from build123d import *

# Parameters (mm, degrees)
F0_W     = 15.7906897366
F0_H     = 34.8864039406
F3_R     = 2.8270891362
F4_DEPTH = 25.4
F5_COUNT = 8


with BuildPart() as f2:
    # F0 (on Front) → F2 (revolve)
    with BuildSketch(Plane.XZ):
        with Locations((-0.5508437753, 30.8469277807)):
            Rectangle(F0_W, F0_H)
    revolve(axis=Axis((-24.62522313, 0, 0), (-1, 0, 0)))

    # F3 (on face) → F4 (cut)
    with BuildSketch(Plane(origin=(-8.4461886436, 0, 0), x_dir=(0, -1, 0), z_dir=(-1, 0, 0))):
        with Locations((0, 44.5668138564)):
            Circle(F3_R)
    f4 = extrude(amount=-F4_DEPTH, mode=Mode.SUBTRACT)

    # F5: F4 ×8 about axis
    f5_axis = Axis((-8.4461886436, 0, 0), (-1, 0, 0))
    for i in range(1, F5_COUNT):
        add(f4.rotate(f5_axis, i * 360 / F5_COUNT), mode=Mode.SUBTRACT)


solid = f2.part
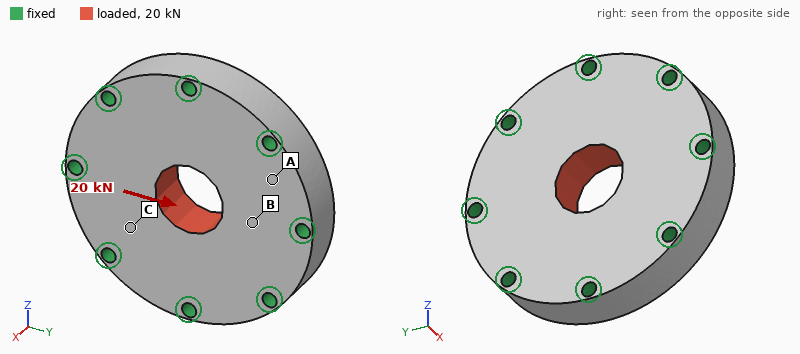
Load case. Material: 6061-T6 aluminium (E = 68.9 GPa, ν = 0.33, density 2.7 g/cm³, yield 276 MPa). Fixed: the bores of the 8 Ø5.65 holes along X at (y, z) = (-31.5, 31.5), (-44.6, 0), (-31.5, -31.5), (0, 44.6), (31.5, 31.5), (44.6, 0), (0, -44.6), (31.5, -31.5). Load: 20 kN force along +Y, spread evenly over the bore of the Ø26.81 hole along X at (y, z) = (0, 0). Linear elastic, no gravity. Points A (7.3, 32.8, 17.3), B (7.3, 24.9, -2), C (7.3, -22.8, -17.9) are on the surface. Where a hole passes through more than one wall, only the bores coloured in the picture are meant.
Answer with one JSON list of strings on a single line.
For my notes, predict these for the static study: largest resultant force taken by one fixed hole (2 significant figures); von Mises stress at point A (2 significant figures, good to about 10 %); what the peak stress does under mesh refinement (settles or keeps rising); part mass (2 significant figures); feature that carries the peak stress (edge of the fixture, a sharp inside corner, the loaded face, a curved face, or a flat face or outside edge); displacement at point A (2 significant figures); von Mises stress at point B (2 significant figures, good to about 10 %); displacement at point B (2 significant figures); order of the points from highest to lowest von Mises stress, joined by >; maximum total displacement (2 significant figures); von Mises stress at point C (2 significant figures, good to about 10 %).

["4.1 kN", "3.4 MPa", "keeps rising", "280 g", "edge of the fixture", "2.9 µm", "14 MPa", "4.3 µm", "B > C > A", "6.8 µm", "9.7 MPa"]
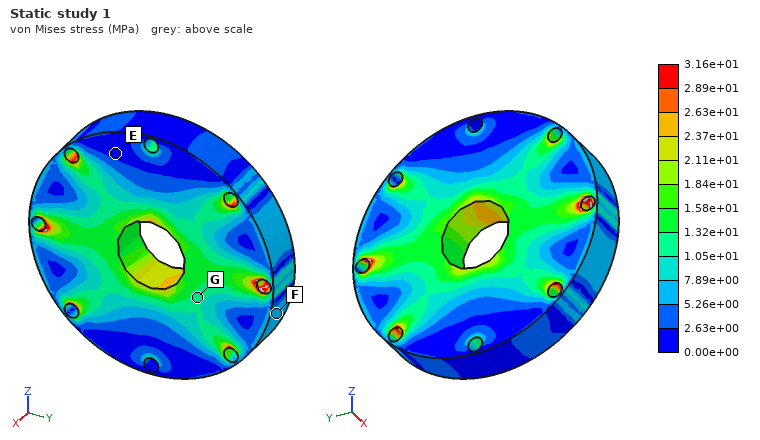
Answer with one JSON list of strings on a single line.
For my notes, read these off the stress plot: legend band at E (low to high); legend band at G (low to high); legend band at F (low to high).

["0.00e+00 to 2.63e+00 MPa", "1.05e+01 to 1.32e+01 MPa", "5.26e+00 to 7.89e+00 MPa"]
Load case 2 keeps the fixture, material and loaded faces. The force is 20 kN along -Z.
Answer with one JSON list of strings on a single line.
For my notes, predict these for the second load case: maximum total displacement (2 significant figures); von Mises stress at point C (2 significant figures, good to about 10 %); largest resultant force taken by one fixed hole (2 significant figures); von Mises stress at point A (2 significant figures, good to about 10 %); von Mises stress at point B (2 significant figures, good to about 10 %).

["6.8 µm", "10 MPa", "4.1 kN", "4.7 MPa", "5.9 MPa"]
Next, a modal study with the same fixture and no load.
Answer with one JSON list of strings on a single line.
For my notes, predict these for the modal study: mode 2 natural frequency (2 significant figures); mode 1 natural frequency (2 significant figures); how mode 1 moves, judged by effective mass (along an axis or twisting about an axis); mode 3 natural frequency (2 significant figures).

["22 kHz", "14 kHz", "along X", "22 kHz"]
